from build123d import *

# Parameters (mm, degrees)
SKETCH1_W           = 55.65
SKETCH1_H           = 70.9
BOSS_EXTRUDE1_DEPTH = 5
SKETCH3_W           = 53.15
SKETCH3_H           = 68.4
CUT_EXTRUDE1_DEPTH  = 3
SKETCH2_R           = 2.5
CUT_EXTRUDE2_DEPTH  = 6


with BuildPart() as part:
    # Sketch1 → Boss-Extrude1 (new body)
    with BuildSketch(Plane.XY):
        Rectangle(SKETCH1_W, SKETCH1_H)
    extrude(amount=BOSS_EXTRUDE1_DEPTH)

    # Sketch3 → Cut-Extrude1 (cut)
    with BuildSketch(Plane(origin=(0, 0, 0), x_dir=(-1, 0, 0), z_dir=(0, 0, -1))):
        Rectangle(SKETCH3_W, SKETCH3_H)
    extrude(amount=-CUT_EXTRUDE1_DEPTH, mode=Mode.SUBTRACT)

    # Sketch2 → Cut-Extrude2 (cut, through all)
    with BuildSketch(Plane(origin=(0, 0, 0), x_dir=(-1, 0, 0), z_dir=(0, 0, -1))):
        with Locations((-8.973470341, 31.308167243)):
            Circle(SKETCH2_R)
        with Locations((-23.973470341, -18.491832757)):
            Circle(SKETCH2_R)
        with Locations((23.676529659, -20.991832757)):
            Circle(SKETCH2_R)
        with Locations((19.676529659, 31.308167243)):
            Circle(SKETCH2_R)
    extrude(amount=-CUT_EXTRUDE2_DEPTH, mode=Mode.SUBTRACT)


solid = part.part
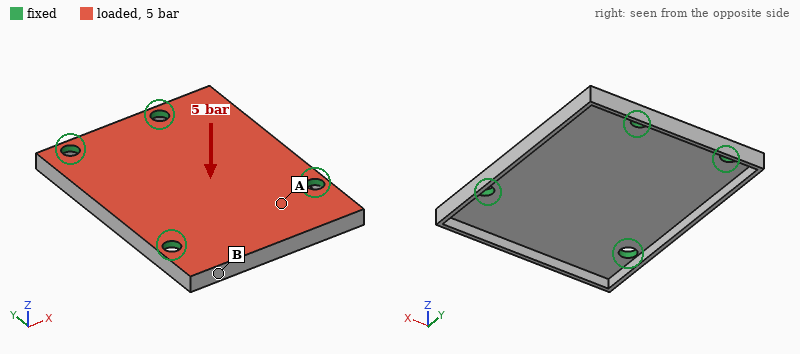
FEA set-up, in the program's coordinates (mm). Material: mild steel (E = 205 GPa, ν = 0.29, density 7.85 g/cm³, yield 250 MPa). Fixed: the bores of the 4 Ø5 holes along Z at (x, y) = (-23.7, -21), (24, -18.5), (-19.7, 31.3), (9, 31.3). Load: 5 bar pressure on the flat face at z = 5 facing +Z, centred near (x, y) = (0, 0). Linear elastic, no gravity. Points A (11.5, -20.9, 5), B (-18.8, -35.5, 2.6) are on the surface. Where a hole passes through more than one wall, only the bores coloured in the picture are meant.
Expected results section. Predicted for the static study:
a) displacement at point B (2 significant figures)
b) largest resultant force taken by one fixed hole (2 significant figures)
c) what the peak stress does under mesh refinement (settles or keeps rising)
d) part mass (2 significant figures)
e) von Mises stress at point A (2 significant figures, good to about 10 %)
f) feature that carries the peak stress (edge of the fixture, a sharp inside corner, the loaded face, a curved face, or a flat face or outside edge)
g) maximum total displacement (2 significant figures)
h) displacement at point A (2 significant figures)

18 µm
590 N
keeps rising
68 g
57 MPa
edge of the fixture
79 µm
30 µm
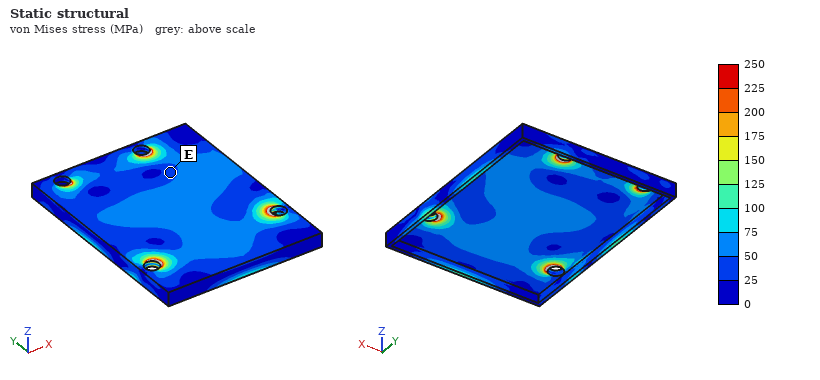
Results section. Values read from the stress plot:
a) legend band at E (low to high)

25 to 50 MPa
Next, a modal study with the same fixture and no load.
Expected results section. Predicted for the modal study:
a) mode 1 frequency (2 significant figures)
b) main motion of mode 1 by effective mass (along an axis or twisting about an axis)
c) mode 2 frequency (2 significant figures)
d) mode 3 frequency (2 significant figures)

3900 Hz
along Z
4600 Hz
5100 Hz
